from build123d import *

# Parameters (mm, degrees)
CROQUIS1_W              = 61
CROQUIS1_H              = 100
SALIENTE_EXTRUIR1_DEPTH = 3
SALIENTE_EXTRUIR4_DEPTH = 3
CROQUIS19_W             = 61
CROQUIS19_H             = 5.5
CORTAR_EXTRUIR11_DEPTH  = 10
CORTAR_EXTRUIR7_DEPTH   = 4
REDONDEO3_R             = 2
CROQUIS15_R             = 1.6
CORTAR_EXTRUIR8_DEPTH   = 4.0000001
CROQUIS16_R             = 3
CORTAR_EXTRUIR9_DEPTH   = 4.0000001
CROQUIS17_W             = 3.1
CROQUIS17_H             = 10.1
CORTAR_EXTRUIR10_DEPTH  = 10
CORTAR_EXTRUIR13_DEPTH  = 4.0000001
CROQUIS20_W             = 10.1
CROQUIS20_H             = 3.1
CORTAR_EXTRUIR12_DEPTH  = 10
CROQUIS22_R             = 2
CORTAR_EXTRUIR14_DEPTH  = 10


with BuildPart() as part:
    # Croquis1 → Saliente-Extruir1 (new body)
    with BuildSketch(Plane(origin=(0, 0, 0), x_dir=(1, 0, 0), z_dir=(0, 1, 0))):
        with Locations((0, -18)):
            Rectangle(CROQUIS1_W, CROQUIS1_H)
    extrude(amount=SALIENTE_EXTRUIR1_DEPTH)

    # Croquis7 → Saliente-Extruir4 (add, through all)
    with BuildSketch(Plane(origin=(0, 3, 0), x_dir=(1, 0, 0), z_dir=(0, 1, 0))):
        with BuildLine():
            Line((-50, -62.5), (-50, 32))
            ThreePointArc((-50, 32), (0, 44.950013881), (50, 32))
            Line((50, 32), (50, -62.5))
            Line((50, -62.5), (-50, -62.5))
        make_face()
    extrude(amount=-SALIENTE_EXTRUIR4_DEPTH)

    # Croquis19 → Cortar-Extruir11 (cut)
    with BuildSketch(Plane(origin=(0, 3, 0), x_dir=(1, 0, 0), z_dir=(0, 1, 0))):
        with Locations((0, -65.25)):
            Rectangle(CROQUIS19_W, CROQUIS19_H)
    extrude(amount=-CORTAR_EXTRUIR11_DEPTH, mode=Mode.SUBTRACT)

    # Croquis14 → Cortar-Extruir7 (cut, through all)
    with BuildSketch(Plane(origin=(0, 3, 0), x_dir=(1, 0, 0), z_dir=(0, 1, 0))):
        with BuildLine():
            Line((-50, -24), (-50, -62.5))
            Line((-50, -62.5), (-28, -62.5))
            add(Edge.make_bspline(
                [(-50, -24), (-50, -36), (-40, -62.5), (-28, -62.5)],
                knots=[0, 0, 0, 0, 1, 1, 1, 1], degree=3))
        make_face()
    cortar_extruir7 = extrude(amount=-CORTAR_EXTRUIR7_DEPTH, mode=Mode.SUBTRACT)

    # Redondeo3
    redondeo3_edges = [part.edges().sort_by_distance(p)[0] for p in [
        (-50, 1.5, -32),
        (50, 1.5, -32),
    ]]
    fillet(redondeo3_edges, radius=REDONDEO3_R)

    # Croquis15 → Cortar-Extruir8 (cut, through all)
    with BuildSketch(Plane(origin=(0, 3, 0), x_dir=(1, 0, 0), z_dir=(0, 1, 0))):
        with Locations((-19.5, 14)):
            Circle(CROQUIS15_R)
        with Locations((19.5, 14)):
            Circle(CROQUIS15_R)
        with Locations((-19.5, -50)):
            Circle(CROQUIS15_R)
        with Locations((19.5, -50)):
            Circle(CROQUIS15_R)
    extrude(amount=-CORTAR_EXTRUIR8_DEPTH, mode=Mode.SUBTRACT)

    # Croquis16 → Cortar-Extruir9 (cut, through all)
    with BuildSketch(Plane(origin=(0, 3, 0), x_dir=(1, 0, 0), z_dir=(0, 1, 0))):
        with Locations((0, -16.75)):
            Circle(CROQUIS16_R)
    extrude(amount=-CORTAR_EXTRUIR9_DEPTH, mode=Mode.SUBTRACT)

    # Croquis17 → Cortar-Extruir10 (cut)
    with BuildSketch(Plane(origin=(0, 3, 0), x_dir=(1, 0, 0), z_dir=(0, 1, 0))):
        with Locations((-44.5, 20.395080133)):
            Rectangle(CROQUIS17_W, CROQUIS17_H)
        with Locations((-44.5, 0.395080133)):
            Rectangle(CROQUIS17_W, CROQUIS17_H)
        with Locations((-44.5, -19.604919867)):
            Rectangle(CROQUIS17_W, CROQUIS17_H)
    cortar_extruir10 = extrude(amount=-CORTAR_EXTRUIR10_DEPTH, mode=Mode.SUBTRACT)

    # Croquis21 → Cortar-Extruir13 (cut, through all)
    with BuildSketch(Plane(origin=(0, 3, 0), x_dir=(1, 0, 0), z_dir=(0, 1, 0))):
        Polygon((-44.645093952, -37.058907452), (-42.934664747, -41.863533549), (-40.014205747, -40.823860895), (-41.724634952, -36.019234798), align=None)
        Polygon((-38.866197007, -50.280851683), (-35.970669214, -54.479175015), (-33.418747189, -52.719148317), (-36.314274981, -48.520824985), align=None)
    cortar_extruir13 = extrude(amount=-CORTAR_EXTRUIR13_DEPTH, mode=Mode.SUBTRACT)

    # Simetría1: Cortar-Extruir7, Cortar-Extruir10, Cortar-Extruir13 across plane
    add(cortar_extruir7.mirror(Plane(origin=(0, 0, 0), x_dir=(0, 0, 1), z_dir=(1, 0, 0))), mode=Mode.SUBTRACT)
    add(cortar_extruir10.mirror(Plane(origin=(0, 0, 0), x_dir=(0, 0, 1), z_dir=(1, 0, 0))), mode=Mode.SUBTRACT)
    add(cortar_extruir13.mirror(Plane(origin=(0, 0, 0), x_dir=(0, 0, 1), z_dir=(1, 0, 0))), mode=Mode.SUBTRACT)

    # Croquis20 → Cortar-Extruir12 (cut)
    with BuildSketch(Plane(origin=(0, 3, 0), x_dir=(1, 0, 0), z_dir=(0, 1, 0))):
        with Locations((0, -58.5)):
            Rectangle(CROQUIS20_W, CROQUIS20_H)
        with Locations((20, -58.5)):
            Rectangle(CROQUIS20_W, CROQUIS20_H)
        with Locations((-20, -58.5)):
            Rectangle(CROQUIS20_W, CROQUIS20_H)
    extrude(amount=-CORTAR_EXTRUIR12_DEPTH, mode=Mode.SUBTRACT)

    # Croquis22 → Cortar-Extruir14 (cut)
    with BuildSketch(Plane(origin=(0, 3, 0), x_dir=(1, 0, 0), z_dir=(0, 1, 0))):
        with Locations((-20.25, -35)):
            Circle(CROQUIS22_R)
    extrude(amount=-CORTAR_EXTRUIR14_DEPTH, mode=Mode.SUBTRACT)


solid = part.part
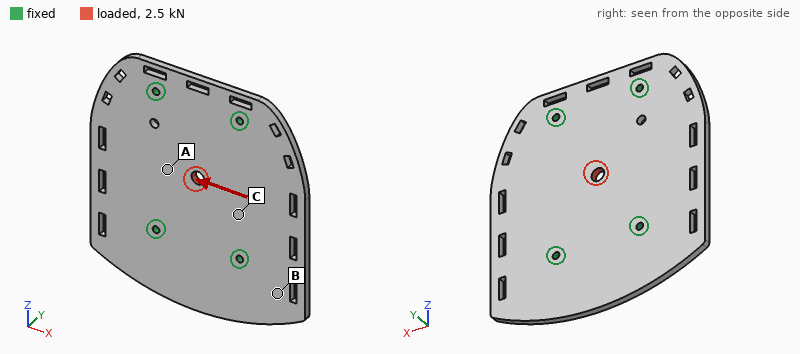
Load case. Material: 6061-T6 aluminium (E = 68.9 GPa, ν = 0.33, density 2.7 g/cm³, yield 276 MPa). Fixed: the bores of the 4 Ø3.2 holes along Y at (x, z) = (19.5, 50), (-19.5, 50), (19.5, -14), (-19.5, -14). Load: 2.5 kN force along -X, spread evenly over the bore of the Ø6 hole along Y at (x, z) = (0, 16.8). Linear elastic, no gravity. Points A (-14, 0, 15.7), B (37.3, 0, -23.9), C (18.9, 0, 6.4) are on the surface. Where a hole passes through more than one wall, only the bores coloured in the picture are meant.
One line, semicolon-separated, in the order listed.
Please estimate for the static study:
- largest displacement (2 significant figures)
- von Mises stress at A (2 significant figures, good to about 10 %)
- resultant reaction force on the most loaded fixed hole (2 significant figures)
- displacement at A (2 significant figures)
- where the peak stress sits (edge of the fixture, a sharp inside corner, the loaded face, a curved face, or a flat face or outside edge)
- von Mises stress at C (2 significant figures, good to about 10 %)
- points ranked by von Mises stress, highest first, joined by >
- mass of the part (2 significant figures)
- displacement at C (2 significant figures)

12 µm; 15 MPa; 680 N; 7.8 µm; the loaded face; 10 MPa; A > C > B; 77 g; 5.8 µm
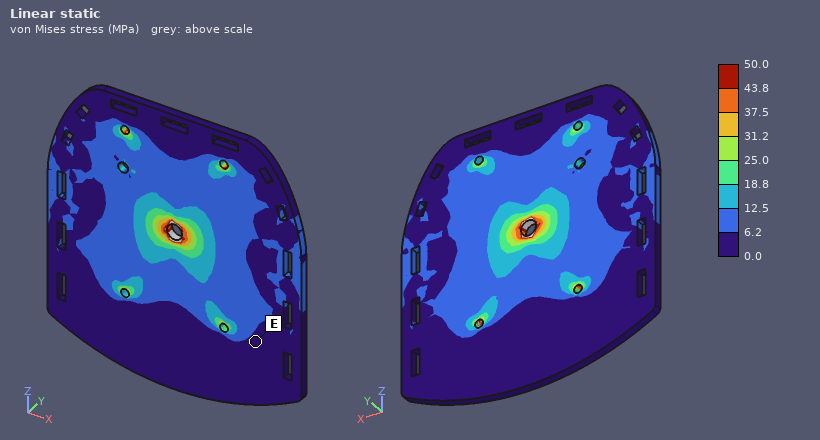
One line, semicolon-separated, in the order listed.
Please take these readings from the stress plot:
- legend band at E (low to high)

0.0 to 6.2 MPa
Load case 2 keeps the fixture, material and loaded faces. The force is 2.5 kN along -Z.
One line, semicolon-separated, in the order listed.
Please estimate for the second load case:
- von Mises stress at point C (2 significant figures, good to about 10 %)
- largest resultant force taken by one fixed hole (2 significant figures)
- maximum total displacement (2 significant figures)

5.7 MPa; 690 N; 9.9 µm
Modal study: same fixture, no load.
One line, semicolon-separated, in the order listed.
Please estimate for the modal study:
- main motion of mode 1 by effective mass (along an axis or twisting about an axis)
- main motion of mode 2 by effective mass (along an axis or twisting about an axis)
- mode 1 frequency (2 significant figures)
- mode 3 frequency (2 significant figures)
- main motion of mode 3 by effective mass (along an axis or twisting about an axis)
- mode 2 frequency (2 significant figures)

along Y; twisting about Z; 2100 Hz; 2500 Hz; along Y; 2200 Hz
